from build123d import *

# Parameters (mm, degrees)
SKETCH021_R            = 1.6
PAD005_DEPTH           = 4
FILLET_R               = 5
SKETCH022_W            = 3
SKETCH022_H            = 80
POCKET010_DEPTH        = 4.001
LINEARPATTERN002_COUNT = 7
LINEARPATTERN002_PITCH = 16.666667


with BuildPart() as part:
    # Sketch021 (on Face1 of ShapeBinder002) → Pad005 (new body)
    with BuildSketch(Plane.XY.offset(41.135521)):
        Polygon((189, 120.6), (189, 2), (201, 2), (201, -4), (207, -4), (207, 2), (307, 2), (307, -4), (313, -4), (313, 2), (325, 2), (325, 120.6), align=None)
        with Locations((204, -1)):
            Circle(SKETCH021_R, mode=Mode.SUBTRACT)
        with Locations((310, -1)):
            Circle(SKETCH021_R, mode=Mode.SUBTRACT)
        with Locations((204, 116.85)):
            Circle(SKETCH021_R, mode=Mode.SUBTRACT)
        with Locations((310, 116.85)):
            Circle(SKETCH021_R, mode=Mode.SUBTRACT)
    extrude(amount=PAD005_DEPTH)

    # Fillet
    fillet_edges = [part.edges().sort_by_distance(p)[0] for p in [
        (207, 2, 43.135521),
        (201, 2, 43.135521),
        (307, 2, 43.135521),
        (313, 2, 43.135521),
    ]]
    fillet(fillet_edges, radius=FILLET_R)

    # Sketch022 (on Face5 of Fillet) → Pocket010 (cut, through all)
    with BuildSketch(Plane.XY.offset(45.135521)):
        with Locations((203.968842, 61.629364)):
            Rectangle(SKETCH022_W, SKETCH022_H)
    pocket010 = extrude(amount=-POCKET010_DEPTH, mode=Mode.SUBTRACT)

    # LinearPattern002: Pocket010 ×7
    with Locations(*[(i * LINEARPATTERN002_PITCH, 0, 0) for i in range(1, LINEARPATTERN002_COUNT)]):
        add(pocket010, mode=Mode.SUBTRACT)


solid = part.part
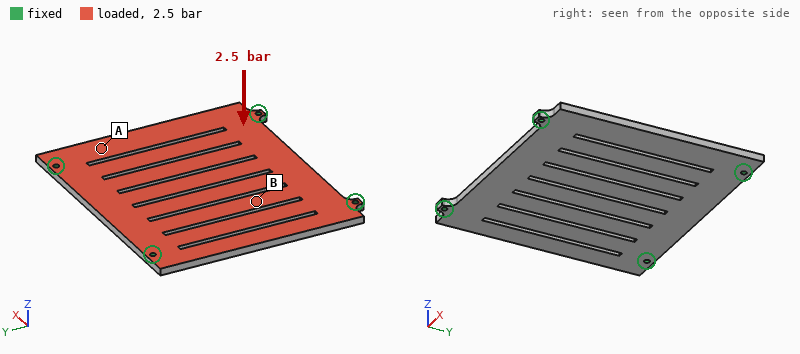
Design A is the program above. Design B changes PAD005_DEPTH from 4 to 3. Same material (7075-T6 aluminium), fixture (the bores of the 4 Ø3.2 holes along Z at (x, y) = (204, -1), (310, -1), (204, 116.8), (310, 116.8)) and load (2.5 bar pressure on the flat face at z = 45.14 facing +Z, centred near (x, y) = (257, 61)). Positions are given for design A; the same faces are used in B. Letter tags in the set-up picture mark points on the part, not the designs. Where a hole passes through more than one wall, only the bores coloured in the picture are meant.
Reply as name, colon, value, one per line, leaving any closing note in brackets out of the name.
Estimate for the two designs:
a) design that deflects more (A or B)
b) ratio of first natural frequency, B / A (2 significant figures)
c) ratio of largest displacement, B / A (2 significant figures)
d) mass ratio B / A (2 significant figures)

design that deflects more: B
ratio of first natural frequency, B / A: 0.76
ratio of largest displacement, B / A: 2.3
mass ratio B / A: 0.75
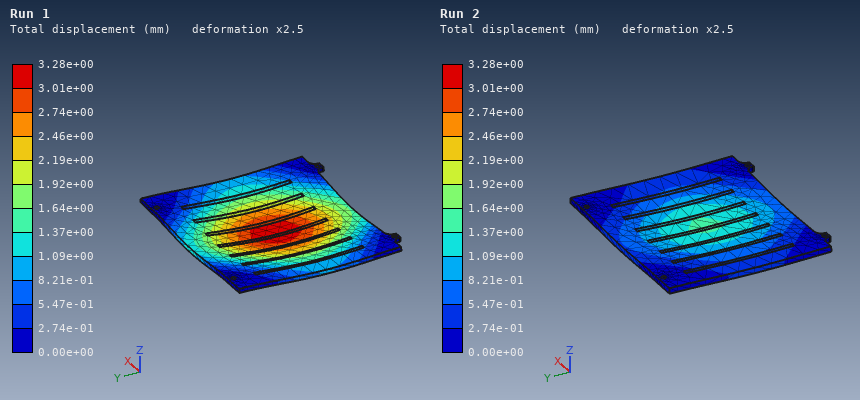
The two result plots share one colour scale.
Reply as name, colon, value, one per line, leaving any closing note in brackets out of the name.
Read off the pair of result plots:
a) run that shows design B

run that shows design B: Run 1
